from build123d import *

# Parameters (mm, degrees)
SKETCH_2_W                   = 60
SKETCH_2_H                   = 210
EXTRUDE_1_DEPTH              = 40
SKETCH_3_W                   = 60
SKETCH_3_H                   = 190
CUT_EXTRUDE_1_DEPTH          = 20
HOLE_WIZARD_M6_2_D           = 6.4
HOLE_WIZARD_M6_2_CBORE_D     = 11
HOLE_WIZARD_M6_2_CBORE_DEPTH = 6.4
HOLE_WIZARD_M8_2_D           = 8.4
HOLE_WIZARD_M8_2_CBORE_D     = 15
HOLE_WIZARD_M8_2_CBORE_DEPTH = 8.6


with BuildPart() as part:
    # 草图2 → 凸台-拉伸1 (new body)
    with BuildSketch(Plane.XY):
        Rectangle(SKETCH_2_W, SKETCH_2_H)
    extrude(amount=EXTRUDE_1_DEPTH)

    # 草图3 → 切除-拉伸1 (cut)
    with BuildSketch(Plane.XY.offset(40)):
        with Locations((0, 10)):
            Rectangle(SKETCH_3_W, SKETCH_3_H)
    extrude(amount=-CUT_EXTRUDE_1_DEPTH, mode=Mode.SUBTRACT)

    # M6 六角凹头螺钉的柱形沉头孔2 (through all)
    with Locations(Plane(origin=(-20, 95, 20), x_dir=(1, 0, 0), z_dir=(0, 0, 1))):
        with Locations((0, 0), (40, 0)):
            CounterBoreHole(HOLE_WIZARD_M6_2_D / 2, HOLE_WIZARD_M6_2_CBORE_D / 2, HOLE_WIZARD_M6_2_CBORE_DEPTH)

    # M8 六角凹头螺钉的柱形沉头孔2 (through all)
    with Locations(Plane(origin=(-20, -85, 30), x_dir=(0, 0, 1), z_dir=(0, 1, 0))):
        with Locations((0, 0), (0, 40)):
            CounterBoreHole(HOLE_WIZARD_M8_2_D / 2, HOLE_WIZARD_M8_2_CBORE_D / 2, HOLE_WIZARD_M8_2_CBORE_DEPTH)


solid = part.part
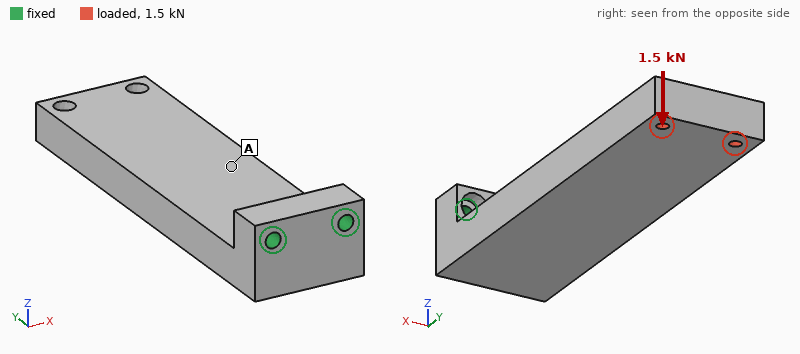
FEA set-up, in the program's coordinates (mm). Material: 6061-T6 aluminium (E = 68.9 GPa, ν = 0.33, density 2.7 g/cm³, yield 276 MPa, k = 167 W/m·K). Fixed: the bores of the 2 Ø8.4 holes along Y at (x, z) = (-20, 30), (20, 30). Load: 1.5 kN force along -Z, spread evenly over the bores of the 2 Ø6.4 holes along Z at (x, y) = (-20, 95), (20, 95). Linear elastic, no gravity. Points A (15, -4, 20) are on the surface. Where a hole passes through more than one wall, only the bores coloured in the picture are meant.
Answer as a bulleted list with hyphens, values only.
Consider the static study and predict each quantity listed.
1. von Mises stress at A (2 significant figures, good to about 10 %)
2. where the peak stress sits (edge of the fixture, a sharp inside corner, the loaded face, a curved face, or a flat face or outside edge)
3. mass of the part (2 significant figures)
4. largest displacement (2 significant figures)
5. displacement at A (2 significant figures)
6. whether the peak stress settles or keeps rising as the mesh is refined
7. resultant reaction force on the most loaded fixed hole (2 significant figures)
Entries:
- 37 MPa
- edge of the fixture
- 730 g
- 2.1 mm
- 0.73 mm
- keeps rising
- 1.3 kN
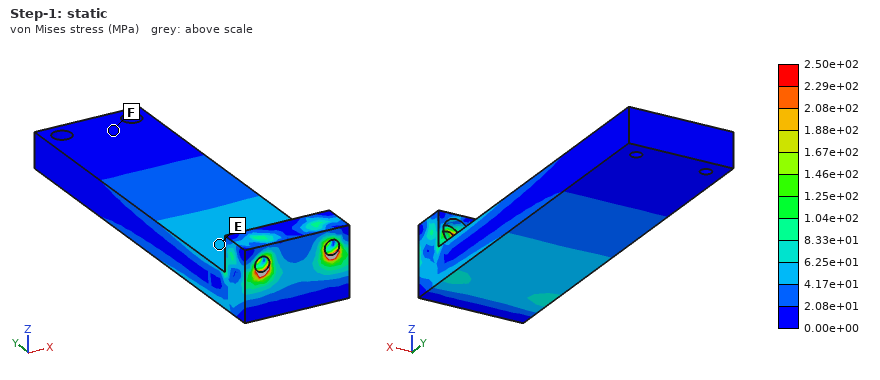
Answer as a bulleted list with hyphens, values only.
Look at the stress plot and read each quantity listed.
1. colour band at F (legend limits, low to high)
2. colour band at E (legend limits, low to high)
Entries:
- 0.00e+00 to 2.08e+01 MPa
- 4.17e+01 to 6.25e+01 MPa
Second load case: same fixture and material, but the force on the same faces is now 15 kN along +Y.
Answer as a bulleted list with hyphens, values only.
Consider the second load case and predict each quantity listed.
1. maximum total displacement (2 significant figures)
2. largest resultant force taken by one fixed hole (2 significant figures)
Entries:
- 1.2 mm
- 7.5 kN
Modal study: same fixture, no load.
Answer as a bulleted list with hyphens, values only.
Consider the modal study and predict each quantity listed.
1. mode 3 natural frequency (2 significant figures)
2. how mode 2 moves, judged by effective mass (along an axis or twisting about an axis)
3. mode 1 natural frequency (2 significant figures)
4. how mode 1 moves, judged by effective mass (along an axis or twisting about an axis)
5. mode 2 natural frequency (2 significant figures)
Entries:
- 1900 Hz
- along X
- 310 Hz
- along Z
- 770 Hz
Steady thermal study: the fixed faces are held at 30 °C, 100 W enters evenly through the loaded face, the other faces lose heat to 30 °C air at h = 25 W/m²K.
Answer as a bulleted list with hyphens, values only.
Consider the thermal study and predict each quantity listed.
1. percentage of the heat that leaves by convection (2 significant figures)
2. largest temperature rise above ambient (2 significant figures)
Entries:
- 36 %
- 82 K
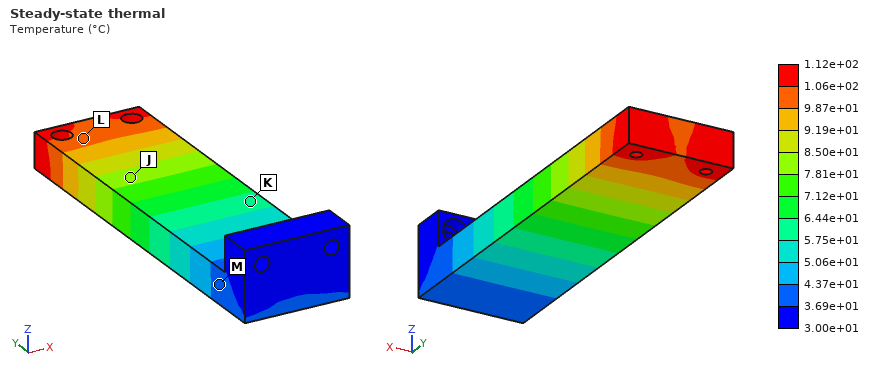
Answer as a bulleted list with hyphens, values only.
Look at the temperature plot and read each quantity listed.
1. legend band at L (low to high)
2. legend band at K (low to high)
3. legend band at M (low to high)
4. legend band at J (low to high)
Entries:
- 9.87e+01 to 1.06e+02 °C
- 5.75e+01 to 6.44e+01 °C
- 3.69e+01 to 4.37e+01 °C
- 7.81e+01 to 8.50e+01 °C
